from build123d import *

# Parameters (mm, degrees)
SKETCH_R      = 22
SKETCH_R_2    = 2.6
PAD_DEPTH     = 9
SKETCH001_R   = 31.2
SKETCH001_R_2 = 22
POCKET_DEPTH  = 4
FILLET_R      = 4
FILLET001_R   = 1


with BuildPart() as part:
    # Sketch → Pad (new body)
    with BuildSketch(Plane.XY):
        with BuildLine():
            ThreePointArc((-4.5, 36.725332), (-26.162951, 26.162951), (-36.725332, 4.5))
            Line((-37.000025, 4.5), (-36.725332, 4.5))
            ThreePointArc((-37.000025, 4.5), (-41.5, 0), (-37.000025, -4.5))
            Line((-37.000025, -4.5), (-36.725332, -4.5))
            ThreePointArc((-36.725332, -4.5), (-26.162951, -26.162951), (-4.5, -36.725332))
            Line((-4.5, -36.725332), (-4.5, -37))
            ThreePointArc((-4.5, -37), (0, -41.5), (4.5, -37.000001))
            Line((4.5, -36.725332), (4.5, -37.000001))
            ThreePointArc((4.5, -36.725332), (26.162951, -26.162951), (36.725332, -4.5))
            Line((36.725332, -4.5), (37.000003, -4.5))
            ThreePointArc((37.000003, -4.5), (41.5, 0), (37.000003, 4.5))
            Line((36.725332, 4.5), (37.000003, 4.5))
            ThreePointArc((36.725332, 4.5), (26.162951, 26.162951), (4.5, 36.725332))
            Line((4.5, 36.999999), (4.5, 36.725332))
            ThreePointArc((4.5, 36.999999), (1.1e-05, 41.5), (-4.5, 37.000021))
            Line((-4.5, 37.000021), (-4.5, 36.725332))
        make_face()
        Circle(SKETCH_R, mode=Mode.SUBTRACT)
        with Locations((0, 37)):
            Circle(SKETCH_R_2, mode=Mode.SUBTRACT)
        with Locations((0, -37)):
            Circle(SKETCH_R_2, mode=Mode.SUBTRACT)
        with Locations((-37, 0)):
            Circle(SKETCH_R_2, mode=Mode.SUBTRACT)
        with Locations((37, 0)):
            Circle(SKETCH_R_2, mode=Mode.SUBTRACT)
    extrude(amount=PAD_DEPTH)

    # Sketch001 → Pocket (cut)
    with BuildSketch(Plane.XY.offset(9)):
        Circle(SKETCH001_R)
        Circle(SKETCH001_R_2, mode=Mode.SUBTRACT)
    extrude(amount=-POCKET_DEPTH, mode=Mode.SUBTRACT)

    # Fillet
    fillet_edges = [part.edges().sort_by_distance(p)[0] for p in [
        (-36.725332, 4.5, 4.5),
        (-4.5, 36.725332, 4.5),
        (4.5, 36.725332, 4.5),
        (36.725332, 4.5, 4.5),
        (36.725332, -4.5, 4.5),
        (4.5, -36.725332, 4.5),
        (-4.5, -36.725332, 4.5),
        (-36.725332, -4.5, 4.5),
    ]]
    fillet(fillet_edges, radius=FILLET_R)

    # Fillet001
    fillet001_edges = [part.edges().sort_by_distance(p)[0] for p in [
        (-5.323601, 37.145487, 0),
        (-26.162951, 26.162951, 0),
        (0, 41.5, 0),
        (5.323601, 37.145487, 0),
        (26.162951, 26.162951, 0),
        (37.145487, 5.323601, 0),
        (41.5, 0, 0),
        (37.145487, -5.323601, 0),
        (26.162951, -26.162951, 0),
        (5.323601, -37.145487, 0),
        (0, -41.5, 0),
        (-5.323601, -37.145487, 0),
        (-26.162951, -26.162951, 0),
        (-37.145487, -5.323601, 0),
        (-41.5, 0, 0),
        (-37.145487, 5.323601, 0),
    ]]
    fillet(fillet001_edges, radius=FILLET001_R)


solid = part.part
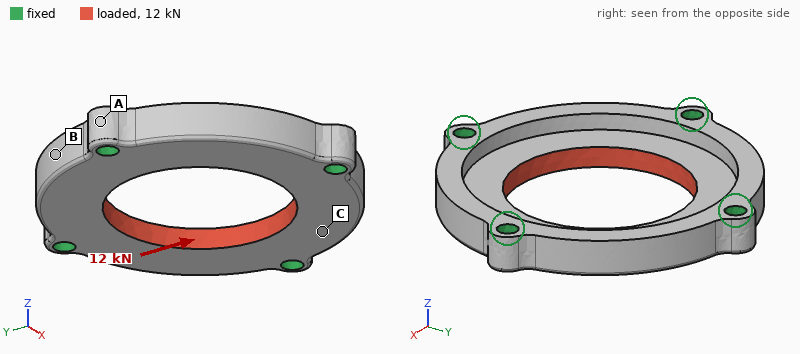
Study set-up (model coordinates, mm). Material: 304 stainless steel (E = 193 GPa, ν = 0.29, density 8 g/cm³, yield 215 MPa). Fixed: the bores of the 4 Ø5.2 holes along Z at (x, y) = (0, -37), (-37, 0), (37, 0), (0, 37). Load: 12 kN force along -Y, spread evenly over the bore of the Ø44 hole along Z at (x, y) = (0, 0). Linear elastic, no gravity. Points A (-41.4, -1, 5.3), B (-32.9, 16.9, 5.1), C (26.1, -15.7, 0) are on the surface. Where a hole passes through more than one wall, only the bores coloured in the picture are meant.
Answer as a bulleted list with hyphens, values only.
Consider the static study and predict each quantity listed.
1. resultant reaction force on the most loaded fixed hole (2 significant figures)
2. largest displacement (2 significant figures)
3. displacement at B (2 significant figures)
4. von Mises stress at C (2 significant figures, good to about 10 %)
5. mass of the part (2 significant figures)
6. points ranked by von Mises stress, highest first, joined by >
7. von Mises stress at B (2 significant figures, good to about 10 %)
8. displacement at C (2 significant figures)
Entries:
- 3.2 kN
- 6.7 µm
- 3.6 µm
- 16 MPa
- 150 g
- B > C > A
- 24 MPa
- 5.3 µm
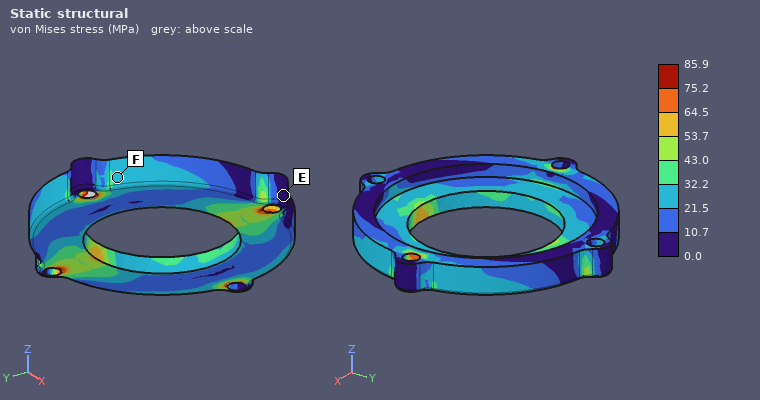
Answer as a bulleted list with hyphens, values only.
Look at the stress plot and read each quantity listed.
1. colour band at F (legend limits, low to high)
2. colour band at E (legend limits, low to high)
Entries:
- 21.5 to 32.2 MPa
- 0.0 to 10.7 MPa
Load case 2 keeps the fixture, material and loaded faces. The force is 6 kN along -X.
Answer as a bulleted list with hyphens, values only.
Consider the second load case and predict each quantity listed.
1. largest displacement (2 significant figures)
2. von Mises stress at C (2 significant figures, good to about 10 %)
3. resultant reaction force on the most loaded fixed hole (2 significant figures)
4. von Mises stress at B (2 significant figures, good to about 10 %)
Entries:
- 3.3 µm
- 11 MPa
- 1.6 kN
- 6.3 MPa
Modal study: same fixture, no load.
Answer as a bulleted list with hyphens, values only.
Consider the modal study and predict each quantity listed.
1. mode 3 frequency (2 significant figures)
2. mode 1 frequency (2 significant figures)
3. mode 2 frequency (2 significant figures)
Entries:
- 13 kHz
- 13 kHz
- 13 kHz
